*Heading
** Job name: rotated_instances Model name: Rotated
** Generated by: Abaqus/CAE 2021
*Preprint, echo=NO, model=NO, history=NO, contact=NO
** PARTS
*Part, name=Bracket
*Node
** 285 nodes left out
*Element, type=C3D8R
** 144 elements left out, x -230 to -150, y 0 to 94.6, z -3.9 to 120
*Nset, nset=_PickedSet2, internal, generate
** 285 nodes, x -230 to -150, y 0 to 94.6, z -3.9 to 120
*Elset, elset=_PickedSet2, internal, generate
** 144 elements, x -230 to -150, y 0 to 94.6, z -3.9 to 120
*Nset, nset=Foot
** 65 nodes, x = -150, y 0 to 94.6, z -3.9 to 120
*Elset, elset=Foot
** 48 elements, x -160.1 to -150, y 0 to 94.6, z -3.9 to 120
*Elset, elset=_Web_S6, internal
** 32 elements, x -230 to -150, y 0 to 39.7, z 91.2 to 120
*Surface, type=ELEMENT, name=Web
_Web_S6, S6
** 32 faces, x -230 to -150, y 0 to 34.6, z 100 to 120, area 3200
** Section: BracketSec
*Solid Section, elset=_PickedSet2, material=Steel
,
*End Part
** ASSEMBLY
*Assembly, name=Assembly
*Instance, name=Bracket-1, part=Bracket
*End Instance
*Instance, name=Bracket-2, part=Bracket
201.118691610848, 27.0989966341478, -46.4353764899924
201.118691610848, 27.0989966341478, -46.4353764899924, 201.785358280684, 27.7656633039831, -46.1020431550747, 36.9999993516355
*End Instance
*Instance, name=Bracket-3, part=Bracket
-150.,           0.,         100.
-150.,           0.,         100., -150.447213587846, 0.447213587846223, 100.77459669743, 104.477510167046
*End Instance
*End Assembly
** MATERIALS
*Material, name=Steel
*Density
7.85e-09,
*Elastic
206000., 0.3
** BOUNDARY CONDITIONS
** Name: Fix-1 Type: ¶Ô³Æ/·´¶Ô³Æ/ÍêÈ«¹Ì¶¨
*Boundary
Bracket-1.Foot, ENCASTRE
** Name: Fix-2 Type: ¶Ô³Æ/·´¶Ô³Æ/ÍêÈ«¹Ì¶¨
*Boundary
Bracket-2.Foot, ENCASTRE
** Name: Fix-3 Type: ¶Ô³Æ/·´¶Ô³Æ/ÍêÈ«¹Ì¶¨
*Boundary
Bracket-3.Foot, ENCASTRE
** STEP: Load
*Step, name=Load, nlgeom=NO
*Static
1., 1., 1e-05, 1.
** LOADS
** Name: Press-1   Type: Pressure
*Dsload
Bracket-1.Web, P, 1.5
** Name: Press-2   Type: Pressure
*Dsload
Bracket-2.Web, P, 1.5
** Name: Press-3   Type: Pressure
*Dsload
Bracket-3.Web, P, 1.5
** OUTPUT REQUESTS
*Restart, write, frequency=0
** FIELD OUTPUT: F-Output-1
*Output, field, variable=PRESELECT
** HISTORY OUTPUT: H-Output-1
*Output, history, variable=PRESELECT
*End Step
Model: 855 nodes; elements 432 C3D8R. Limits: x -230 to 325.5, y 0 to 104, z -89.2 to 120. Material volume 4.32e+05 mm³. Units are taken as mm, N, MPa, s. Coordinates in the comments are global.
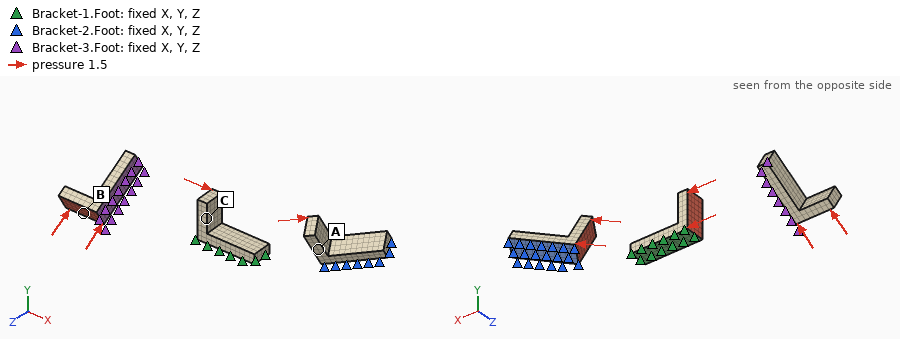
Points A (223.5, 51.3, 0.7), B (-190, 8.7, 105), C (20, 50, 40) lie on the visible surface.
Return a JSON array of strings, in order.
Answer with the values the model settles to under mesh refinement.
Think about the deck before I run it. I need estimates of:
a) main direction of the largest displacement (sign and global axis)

["+X"]
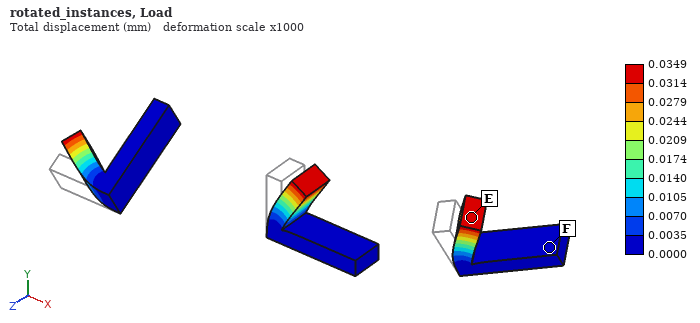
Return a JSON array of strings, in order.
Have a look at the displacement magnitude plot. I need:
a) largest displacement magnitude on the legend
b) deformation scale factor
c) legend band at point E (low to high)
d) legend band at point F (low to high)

["0.0349 mm", "1000", "0.0314 to 0.0349 mm", "0.0000 to 0.0035 mm"]
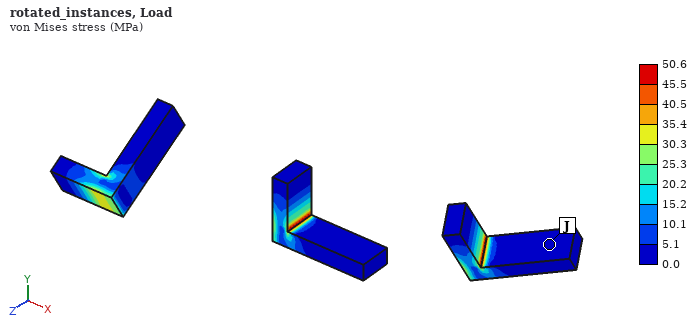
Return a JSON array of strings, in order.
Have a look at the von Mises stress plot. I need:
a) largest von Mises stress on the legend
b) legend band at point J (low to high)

["50.6 MPa", "0.0 to 5.1 MPa"]
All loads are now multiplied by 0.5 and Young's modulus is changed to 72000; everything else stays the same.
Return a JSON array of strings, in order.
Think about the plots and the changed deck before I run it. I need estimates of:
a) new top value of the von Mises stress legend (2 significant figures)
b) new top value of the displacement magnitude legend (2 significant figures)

["25 MPa", "0.050 mm"]
